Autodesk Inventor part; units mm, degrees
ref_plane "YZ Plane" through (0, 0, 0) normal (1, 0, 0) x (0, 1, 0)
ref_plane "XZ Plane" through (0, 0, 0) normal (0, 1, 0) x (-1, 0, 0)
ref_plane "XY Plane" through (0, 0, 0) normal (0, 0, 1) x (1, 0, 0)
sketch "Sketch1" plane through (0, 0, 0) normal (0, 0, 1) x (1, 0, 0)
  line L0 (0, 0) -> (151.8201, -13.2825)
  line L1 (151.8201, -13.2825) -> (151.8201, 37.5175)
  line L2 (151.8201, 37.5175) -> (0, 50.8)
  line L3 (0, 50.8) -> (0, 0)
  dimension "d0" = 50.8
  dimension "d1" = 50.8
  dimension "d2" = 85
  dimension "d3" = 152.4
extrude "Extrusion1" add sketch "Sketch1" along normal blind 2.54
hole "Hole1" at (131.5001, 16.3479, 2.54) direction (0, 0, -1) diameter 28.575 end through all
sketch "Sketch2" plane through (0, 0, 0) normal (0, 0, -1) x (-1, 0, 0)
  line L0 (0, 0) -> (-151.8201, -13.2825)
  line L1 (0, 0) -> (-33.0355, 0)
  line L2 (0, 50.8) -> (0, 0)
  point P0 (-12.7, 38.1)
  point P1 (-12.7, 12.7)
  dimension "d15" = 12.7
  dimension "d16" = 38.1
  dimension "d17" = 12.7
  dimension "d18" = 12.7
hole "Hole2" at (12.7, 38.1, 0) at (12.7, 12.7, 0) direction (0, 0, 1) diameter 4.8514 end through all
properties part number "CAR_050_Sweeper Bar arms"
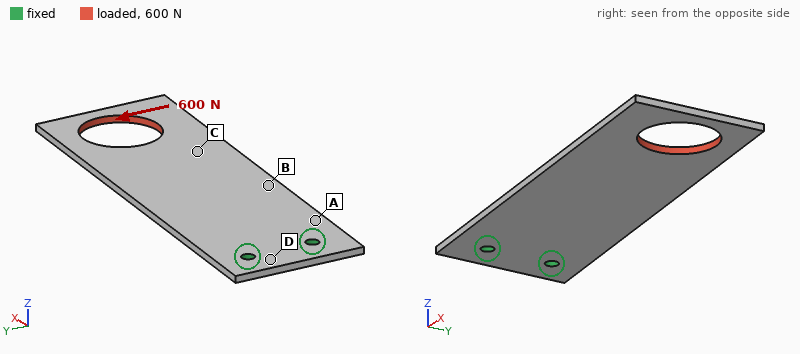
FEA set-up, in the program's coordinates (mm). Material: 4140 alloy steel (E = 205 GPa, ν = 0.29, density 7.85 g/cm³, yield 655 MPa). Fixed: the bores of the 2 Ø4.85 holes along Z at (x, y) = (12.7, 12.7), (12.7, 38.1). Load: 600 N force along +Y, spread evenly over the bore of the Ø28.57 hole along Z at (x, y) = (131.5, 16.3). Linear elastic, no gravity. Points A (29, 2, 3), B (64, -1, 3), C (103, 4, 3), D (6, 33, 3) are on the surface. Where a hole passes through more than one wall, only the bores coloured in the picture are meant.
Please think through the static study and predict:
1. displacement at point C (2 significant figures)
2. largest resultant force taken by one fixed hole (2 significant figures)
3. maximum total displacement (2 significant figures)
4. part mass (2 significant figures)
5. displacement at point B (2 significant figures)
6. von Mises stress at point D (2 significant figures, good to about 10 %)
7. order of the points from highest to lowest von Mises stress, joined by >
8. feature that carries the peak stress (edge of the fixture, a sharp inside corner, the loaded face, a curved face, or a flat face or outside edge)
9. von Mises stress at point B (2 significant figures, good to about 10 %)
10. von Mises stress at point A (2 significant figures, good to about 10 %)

0.059 mm
2.6 kN
0.12 mm
140 g
0.030 mm
20 MPa
A > B > D > C
edge of the fixture
30 MPa
41 MPa
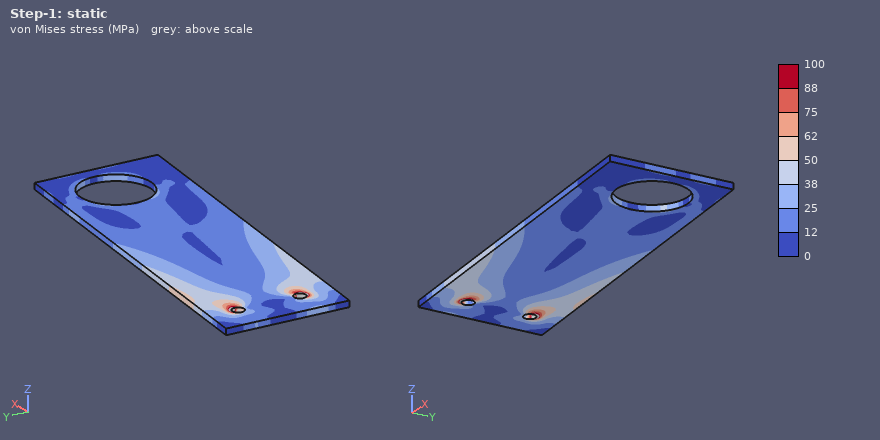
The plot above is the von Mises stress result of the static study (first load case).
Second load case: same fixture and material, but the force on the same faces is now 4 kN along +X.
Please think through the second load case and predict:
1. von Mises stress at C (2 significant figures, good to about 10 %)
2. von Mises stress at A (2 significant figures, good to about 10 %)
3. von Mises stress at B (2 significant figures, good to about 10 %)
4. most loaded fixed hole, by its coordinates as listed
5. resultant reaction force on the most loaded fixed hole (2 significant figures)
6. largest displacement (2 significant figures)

33 MPa
45 MPa
41 MPa
(12.7, 12.7)
3.3 kN
55 µm
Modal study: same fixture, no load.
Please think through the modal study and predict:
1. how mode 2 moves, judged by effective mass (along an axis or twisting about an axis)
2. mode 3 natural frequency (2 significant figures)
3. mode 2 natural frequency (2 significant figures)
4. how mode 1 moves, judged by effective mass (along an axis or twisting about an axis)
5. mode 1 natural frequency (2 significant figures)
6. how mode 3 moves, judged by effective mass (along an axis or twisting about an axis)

twisting about X
690 Hz
610 Hz
along Z
120 Hz
along Z
